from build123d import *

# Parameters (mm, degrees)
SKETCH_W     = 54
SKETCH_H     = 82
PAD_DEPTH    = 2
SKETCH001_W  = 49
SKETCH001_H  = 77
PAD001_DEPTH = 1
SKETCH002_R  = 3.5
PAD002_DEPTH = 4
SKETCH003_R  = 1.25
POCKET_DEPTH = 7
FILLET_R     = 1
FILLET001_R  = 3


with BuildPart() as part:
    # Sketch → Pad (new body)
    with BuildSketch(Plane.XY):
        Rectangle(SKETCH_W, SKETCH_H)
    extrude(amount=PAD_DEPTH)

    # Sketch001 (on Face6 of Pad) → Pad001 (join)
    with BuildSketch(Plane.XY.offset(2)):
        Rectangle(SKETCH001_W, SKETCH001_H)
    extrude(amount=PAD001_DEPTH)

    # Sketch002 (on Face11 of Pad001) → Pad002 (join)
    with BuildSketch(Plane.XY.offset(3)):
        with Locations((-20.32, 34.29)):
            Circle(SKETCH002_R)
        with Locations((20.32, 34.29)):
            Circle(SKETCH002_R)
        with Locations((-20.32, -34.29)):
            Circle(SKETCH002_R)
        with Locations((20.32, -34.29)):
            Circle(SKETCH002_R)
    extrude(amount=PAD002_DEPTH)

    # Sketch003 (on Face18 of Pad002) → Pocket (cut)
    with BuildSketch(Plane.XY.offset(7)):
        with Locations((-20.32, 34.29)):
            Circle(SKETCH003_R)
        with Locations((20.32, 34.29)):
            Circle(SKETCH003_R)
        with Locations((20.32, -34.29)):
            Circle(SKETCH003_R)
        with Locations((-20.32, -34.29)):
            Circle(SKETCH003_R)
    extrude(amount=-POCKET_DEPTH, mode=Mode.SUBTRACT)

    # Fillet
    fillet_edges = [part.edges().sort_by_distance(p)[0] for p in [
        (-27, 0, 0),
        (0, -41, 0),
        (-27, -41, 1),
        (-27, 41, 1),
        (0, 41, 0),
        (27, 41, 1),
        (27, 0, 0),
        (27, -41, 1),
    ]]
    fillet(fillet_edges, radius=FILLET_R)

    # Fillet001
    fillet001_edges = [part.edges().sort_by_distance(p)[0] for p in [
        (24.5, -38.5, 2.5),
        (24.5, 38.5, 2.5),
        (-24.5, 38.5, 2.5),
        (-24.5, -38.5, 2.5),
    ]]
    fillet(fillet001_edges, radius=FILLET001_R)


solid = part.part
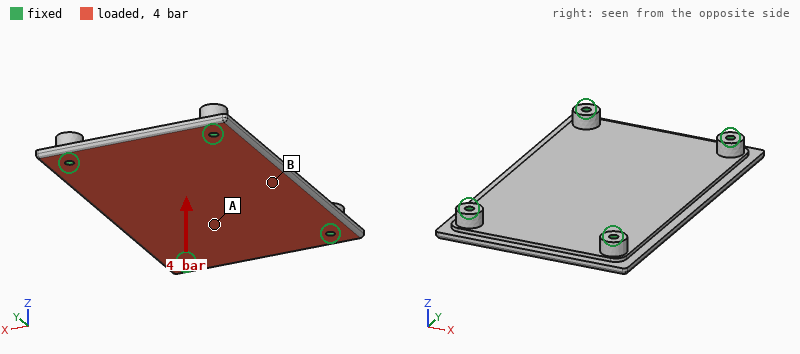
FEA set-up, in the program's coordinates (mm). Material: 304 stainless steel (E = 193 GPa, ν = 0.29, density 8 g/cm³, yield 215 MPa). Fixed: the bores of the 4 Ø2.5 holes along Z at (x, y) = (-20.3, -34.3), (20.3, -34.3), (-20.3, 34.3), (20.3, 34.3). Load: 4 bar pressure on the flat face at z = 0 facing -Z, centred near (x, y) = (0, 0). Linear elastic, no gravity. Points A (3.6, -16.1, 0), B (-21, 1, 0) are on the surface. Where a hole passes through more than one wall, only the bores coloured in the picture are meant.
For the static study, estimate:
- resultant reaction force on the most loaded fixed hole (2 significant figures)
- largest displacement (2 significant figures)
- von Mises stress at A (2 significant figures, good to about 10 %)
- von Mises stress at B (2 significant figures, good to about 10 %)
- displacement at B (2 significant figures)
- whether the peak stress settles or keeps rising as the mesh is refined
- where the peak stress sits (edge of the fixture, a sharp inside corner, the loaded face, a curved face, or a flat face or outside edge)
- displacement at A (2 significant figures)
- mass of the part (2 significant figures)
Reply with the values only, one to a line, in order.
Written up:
430 N
66 µm
26 MPa
59 MPa
62 µm
keeps rising
edge of the fixture
47 µm
100 g
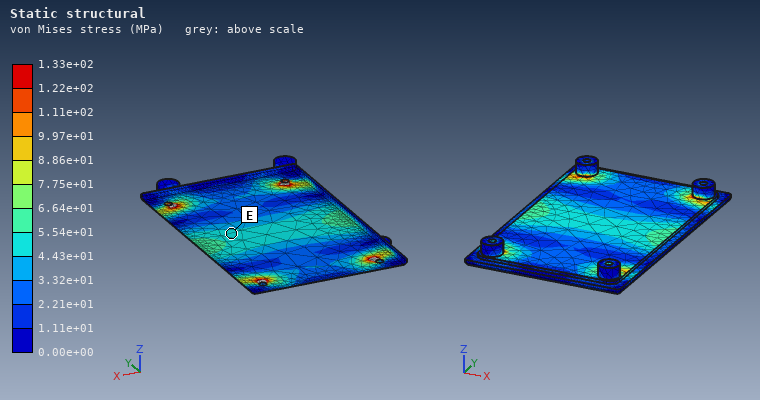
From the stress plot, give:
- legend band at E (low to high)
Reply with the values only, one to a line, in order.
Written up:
4.43e+01 to 5.54e+01 MPa
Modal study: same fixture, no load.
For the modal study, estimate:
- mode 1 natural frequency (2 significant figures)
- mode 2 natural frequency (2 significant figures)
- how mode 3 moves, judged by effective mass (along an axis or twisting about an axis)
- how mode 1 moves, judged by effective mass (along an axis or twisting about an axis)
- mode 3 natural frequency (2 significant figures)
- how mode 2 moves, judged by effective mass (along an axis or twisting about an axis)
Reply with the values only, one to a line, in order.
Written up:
2900 Hz
4300 Hz
twisting about X
along Z
7400 Hz
twisting about Y
